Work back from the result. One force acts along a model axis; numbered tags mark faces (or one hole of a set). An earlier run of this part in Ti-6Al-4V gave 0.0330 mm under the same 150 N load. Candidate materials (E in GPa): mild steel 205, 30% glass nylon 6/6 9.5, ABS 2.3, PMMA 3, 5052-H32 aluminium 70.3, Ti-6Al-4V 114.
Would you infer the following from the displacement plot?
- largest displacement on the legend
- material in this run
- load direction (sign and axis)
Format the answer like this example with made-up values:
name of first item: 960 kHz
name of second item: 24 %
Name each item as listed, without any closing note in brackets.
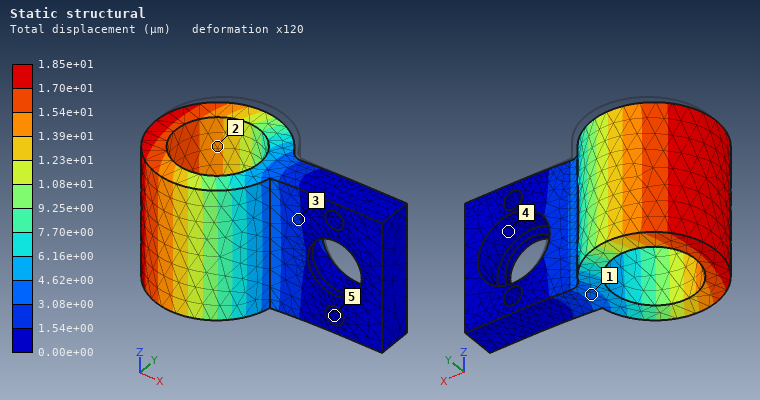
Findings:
largest displacement on the legend: 1.85e+01 µm
material in this run: mild steel
load direction: -Y
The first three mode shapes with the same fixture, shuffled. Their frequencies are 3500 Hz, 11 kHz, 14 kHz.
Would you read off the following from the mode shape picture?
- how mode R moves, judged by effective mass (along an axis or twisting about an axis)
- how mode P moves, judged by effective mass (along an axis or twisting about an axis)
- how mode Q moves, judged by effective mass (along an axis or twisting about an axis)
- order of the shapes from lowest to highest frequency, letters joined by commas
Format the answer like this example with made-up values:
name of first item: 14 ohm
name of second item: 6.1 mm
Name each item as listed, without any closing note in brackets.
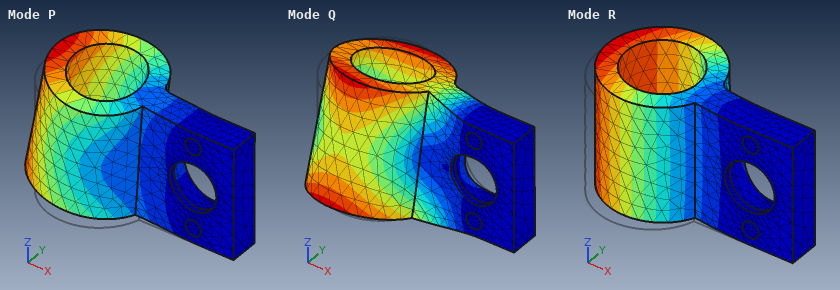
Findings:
how mode R moves, judged by effective mass: along Y
how mode P moves, judged by effective mass: along Z
how mode Q moves, judged by effective mass: twisting about X
order of the shapes from lowest to highest frequency, letters joined by commas: R, P, Q
